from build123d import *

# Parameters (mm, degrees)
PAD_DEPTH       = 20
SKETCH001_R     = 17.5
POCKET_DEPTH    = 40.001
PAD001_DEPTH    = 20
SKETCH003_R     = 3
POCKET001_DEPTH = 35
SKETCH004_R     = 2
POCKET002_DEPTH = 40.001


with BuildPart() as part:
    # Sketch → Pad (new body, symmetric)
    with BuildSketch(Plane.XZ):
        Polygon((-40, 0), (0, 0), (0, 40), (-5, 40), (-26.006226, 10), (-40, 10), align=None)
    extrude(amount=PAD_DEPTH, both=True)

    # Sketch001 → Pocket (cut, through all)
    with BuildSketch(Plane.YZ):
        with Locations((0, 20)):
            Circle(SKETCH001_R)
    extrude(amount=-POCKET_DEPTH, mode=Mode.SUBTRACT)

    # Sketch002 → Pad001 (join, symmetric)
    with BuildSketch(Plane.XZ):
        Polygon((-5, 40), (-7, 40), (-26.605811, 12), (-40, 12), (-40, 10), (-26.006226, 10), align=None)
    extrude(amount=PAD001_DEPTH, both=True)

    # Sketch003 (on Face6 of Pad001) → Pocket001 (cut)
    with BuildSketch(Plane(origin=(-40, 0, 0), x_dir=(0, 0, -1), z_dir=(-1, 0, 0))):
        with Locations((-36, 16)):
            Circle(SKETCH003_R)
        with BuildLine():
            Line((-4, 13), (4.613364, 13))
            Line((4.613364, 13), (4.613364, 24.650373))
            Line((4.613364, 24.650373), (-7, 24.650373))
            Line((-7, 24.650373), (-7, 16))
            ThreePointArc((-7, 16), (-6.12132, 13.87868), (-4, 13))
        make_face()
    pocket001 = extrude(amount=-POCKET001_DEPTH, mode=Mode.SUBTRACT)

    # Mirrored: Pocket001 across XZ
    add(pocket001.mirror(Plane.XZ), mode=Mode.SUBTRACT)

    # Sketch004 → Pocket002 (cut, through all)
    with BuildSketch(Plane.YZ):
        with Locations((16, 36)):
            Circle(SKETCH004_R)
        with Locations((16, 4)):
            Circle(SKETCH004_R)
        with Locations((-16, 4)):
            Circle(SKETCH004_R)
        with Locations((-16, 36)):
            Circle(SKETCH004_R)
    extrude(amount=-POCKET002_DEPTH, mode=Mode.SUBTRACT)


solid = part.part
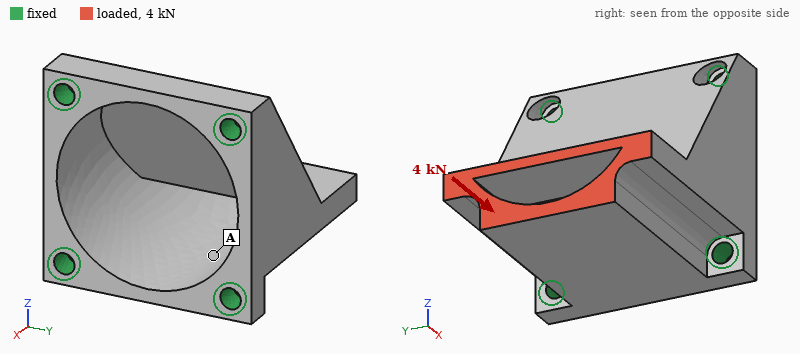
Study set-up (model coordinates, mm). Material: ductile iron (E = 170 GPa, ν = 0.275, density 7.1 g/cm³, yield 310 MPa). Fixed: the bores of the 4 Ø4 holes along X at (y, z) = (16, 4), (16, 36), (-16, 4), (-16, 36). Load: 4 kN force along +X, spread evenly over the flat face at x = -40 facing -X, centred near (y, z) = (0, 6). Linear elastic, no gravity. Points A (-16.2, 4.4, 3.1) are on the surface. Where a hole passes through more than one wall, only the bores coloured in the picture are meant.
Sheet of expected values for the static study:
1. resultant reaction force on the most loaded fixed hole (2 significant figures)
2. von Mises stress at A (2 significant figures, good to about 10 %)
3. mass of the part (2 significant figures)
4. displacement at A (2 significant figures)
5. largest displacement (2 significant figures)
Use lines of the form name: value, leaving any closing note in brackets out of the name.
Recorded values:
resultant reaction force on the most loaded fixed hole: 1.9 kN
von Mises stress at A: 17 MPa
mass of the part: 100 g
displacement at A: 4.3 µm
largest displacement: 12 µm
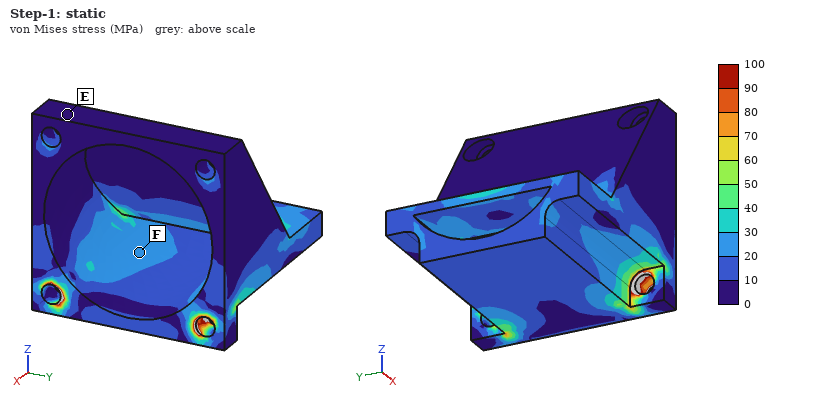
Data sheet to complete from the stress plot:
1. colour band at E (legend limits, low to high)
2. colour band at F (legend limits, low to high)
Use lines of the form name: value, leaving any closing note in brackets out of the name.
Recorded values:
colour band at E: 0 to 10 MPa
colour band at F: 20 to 30 MPa
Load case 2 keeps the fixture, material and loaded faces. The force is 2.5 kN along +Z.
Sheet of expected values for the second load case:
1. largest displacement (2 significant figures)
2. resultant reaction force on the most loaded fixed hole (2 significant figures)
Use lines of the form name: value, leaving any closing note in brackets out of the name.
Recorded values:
largest displacement: 0.11 mm
resultant reaction force on the most loaded fixed hole: 1.9 kN
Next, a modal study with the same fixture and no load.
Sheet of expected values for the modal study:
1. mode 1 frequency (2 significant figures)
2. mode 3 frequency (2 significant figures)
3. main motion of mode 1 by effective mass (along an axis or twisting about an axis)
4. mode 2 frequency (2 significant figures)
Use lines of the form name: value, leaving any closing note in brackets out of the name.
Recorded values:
mode 1 frequency: 9200 Hz
mode 3 frequency: 11 kHz
main motion of mode 1 by effective mass: along Z
mode 2 frequency: 11 kHz
